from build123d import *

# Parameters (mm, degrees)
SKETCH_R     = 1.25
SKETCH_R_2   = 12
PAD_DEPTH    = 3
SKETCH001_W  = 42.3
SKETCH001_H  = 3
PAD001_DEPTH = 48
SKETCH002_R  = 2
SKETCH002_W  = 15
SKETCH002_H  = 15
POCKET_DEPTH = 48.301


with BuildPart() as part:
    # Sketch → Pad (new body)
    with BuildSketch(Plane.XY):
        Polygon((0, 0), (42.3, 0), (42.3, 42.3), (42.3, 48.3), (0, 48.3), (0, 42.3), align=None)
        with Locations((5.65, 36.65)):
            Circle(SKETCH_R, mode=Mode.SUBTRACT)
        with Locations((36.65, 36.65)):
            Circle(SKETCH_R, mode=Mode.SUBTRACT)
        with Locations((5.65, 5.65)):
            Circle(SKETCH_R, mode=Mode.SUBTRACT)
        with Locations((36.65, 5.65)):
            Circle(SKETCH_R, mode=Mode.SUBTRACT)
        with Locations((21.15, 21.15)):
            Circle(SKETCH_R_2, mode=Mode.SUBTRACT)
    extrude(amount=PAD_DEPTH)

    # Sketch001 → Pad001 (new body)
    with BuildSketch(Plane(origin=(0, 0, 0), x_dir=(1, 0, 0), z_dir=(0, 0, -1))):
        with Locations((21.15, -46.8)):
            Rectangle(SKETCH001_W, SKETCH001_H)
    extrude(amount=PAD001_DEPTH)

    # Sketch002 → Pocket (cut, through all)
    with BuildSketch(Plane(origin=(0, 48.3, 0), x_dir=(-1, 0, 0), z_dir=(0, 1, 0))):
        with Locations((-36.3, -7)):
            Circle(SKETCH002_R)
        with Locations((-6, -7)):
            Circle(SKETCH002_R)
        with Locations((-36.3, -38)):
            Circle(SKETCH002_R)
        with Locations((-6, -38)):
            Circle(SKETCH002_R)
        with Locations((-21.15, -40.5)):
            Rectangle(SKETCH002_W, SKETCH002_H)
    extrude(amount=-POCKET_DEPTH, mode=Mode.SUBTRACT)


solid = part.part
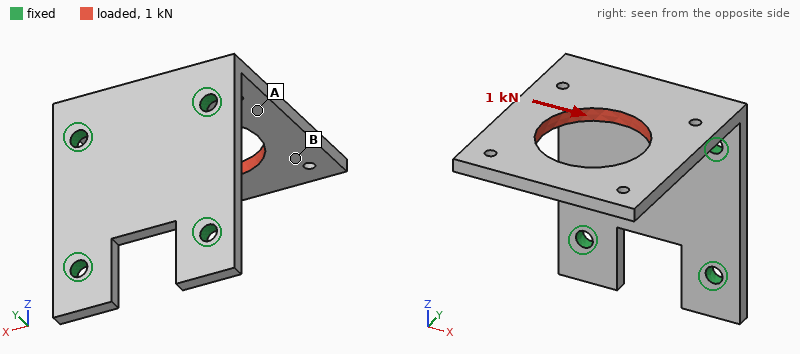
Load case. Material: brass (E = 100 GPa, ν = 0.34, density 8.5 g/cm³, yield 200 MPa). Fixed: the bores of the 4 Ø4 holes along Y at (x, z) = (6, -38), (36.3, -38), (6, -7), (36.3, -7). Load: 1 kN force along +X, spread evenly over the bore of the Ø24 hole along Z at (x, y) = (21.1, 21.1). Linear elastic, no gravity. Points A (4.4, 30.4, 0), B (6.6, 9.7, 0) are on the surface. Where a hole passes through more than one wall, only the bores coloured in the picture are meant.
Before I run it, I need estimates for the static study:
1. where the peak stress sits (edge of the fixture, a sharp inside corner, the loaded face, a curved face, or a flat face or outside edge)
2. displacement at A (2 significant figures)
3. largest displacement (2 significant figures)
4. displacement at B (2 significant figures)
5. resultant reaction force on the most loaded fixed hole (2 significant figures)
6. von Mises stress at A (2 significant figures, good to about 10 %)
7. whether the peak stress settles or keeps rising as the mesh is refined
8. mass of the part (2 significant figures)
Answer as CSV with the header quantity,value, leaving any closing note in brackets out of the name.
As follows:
quantity,value
where the peak stress sits,edge of the fixture
displacement at A,0.066 mm
largest displacement,0.15 mm
displacement at B,0.11 mm
resultant reaction force on the most loaded fixed hole,980 N
von Mises stress at A,34 MPa
whether the peak stress settles or keeps rising as the mesh is refined,keeps rising
mass of the part,85 g
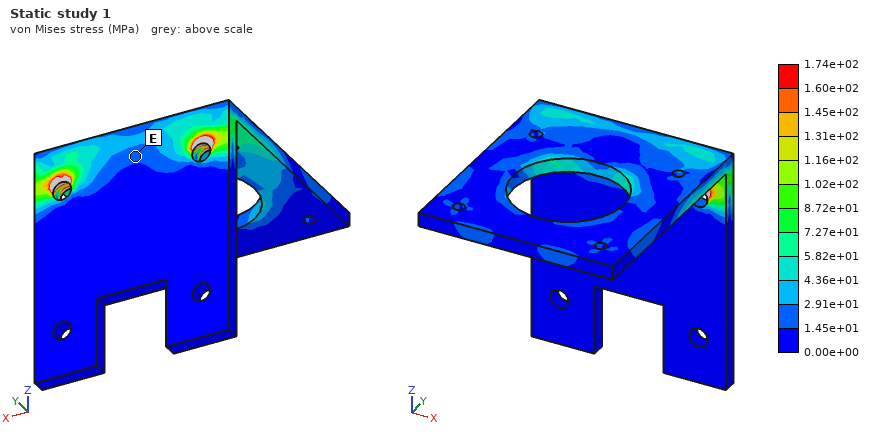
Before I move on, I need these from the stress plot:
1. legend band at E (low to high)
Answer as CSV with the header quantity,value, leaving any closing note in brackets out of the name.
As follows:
quantity,value
legend band at E,1.45e+01 to 2.91e+01 MPa
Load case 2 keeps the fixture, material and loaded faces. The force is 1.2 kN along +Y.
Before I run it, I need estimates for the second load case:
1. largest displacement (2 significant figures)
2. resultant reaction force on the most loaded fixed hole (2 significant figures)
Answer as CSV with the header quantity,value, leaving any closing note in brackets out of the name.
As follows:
quantity,value
largest displacement,0.21 mm
resultant reaction force on the most loaded fixed hole,620 N
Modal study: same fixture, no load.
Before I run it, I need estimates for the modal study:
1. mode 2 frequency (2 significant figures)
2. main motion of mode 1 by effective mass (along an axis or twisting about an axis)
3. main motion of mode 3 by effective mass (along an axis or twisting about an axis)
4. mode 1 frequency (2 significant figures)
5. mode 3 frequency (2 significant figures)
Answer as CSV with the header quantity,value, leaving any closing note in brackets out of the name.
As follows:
quantity,value
mode 2 frequency,1600 Hz
main motion of mode 1 by effective mass,along Z
main motion of mode 3 by effective mass,along X
mode 1 frequency,610 Hz
mode 3 frequency,2900 Hz
